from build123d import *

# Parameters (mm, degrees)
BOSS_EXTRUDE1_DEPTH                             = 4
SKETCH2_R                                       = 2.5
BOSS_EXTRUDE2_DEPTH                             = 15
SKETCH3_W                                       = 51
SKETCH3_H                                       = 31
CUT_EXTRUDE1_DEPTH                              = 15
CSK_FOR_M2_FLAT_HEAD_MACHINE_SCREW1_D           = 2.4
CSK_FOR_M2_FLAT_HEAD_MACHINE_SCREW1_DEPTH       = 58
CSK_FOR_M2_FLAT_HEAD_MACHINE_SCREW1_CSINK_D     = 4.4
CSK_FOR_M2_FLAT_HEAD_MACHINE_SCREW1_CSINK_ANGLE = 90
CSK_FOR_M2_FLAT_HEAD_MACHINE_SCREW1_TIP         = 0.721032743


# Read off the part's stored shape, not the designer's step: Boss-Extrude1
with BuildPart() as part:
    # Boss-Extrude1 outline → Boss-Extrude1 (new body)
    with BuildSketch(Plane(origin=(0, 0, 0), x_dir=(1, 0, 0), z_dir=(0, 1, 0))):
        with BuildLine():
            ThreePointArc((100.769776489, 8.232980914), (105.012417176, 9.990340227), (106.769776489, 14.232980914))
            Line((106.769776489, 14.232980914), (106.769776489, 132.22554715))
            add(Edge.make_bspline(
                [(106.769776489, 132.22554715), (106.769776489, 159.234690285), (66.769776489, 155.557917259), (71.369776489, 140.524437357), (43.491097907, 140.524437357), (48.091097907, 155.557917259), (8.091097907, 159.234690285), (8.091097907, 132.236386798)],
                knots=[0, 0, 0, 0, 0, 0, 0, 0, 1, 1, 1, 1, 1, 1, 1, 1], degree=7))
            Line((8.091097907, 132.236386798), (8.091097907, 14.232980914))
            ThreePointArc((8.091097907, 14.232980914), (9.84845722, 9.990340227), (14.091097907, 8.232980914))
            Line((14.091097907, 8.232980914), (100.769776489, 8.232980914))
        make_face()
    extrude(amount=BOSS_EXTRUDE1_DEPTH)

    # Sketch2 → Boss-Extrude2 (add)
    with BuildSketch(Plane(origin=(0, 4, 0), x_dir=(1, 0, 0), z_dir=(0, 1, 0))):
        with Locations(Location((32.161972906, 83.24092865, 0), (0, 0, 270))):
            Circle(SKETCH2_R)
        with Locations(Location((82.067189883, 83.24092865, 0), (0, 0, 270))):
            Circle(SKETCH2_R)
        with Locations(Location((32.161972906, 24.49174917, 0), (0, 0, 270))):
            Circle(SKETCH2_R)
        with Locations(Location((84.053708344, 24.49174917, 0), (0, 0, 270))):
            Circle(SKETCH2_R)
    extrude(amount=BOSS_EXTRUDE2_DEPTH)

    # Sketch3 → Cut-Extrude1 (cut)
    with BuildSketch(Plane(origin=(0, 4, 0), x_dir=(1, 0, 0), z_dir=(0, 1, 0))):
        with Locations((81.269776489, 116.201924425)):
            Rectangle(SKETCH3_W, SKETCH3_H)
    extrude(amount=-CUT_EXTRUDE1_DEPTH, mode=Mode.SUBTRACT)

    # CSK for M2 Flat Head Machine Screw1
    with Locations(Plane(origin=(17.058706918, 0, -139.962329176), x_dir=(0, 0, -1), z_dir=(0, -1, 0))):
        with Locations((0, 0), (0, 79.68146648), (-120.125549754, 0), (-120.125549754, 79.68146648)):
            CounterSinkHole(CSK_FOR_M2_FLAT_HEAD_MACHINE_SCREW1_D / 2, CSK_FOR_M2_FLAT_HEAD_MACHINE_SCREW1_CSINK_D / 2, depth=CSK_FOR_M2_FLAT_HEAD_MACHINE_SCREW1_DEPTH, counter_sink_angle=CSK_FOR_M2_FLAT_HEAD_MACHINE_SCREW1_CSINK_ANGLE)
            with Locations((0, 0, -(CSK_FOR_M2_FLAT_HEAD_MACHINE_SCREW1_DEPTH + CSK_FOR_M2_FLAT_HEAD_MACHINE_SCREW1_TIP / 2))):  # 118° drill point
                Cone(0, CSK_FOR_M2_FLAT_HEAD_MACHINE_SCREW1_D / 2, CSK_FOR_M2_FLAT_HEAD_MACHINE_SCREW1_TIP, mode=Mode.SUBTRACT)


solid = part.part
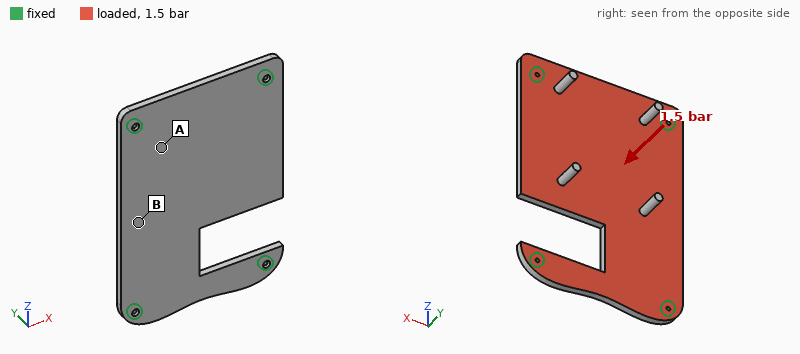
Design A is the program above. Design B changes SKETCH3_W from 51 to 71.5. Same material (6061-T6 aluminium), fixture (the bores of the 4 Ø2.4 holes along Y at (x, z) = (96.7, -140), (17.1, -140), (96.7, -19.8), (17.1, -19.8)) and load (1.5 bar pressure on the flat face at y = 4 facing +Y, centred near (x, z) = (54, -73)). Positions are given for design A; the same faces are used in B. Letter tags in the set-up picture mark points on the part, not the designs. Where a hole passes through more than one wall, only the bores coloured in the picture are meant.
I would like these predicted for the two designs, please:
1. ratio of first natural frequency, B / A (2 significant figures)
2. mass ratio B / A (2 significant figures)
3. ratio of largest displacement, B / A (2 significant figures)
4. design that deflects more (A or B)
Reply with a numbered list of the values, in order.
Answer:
1. 0.93
2. 0.97
3. 1.2
4. B
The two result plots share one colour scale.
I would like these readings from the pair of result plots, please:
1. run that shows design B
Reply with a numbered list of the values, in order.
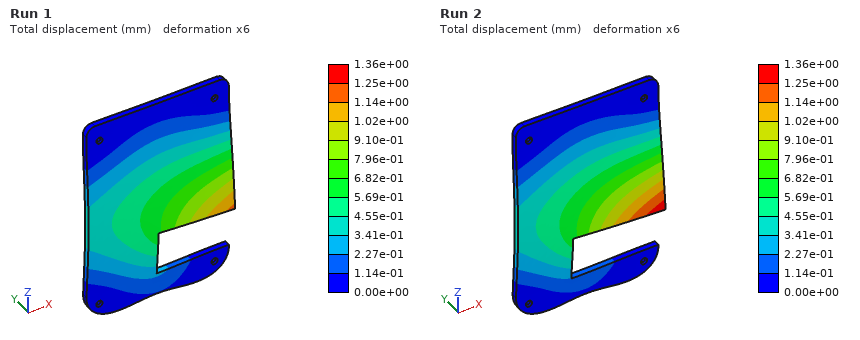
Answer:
1. Run 2
